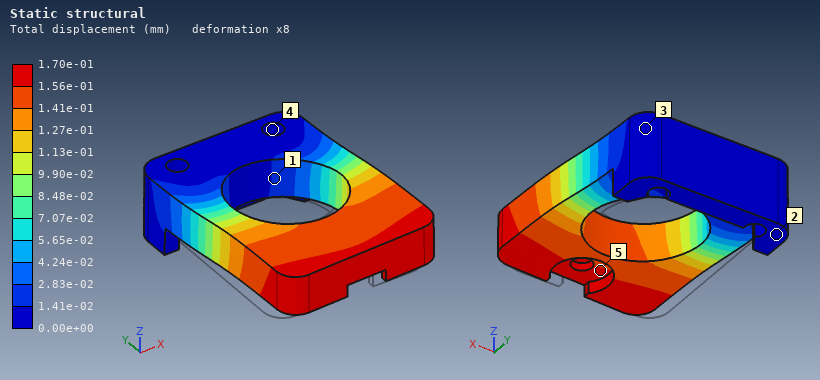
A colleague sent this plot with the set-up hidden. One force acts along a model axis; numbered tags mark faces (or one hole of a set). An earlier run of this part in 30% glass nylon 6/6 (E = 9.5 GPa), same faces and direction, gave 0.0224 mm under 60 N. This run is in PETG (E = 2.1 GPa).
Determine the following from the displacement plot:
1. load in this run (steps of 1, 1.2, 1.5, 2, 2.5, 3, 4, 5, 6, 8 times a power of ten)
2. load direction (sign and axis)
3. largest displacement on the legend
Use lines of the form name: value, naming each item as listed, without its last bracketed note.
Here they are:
load in this run: 100 N
load direction: +X
largest displacement on the legend: 1.70e-01 mm
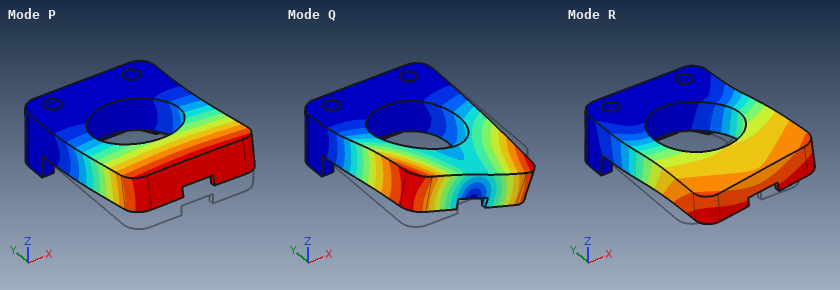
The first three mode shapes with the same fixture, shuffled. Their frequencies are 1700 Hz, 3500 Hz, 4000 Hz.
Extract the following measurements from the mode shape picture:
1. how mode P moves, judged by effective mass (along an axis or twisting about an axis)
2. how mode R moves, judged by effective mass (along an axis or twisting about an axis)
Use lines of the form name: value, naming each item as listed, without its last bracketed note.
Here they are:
how mode P moves, judged by effective mass: along Z
how mode R moves, judged by effective mass: along X
